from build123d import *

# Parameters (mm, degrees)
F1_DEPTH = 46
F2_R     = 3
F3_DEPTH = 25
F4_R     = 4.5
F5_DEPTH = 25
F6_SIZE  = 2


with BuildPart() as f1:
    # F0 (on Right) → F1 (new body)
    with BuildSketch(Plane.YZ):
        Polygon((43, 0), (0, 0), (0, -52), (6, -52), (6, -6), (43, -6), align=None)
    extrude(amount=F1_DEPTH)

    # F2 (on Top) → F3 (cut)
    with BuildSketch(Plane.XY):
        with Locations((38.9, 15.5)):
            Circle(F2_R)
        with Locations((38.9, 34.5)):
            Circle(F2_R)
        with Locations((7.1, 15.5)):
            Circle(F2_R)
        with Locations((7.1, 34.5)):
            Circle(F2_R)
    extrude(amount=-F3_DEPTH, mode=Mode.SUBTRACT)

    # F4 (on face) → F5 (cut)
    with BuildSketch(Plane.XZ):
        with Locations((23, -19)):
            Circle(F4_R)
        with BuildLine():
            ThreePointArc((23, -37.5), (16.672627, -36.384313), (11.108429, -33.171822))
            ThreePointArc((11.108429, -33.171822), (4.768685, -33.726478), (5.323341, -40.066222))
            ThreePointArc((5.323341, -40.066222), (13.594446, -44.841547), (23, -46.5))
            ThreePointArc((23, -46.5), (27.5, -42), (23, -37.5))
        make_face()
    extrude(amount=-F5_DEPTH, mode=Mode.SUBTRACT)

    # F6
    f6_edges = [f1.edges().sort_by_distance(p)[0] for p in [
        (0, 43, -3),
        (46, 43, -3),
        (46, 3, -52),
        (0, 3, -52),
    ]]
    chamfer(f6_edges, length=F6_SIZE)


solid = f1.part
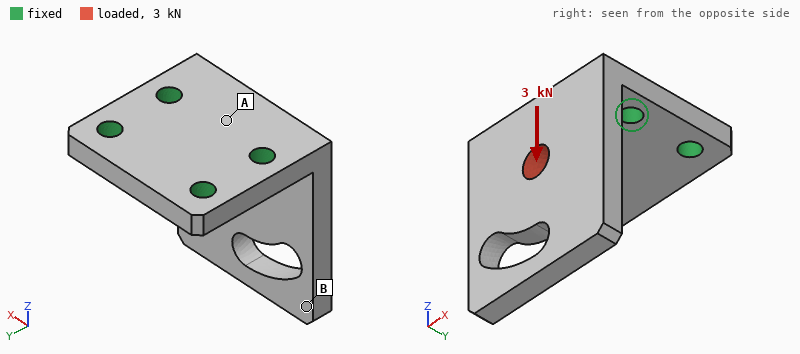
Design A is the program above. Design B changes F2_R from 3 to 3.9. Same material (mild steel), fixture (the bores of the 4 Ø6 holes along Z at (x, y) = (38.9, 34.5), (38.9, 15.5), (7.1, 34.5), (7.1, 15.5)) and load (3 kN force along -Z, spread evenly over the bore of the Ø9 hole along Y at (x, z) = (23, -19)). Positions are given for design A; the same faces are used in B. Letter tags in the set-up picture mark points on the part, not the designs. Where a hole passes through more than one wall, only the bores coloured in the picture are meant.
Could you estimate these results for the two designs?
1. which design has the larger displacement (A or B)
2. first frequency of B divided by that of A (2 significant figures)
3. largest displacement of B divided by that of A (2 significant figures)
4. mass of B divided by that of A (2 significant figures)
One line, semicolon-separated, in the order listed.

A; 1.0; 0.83; 0.98
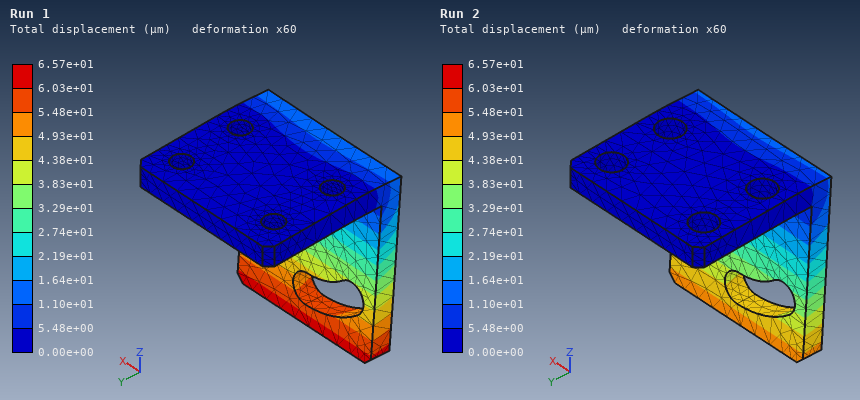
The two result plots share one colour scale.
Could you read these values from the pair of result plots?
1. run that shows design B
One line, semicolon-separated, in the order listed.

Run 2
